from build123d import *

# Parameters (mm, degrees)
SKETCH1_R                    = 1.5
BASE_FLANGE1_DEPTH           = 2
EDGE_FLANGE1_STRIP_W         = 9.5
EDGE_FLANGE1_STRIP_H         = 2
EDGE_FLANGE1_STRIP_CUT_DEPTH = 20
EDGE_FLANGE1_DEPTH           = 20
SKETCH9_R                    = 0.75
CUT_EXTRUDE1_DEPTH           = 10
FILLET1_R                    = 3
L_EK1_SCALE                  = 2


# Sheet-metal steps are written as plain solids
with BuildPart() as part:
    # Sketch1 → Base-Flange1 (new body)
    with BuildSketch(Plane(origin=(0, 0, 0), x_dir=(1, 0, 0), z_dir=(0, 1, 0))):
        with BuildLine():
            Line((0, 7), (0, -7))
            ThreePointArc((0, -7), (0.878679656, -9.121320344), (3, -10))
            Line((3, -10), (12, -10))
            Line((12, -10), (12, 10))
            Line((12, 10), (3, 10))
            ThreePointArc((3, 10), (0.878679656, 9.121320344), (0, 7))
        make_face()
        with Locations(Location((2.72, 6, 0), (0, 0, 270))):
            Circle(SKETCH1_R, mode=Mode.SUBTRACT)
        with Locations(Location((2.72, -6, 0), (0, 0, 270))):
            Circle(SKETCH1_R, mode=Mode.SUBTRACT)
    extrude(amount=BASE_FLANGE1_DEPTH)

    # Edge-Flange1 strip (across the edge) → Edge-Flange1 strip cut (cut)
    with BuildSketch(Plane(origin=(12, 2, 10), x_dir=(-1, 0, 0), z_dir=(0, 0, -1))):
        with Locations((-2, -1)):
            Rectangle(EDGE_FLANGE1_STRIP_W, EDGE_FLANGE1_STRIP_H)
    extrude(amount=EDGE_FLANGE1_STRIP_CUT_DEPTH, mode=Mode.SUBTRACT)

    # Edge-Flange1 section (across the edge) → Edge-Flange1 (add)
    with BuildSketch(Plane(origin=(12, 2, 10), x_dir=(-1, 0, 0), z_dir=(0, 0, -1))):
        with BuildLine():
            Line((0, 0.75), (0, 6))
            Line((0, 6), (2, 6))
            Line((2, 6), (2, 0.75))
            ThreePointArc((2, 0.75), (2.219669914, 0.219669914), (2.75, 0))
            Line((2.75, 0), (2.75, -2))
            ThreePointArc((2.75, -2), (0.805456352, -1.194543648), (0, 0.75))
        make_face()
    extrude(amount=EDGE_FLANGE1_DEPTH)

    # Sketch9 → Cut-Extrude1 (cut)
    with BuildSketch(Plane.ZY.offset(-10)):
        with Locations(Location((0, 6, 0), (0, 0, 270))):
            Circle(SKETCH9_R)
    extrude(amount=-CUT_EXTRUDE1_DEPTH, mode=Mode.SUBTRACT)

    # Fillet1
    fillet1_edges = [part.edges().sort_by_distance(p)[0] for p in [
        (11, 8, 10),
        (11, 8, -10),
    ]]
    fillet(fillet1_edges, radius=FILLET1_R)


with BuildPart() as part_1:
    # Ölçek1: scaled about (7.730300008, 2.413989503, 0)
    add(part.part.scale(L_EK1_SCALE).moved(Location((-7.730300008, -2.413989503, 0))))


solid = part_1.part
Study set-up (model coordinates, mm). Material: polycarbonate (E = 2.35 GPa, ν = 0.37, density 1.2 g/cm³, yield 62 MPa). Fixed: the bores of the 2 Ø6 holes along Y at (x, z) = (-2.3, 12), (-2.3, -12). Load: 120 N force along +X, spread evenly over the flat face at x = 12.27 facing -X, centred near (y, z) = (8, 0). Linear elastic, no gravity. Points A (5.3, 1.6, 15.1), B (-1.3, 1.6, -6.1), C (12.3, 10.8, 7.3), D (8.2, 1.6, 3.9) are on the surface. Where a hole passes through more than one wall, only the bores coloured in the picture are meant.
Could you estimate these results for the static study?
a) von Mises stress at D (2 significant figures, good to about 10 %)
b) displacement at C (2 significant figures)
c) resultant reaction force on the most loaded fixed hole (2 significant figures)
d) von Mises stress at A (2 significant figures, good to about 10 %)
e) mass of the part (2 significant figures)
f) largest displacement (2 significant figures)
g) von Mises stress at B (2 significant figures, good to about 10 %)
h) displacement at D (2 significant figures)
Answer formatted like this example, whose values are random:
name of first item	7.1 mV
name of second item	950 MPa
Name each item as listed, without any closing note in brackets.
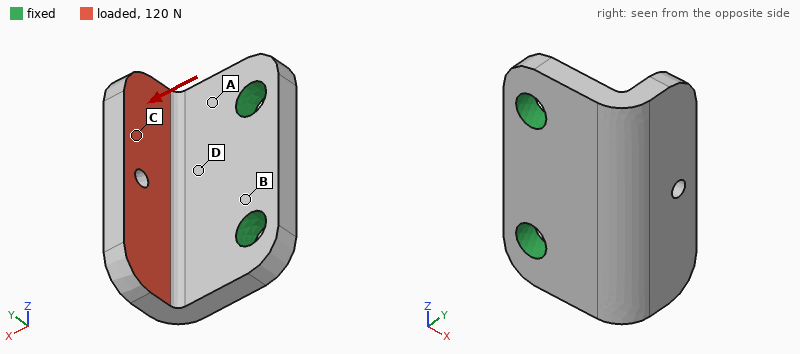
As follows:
von Mises stress at D	8.9 MPa
displacement at C	0.40 mm
resultant reaction force on the most loaded fixed hole	62 N
von Mises stress at A	10.0 MPa
mass of the part	6.2 g
largest displacement	0.55 mm
von Mises stress at B	4.6 MPa
displacement at D	0.096 mm
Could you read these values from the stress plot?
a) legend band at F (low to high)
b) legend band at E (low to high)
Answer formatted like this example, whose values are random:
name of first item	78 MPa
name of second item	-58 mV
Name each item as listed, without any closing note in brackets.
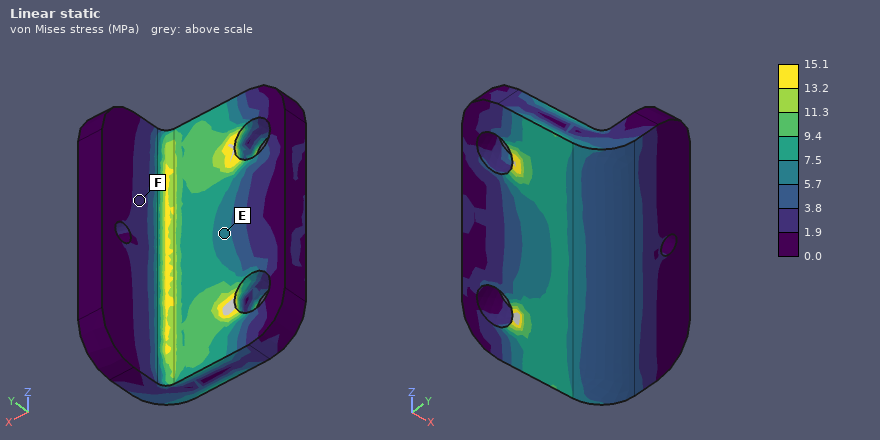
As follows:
legend band at F	1.9 to 3.8 MPa
legend band at E	5.7 to 7.5 MPa
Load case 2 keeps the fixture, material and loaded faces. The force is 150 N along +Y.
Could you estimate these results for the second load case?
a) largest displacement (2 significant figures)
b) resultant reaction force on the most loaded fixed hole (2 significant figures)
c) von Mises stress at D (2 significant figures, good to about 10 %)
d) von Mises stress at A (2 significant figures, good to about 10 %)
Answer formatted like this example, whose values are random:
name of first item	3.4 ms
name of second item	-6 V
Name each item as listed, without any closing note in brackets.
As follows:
largest displacement	0.46 mm
resultant reaction force on the most loaded fixed hole	75 N
von Mises stress at D	4.8 MPa
von Mises stress at A	9.8 MPa
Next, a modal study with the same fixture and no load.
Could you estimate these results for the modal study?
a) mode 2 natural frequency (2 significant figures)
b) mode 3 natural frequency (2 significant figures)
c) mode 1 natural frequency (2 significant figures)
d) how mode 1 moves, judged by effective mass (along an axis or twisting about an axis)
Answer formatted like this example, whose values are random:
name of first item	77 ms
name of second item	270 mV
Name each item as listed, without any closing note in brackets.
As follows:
mode 2 natural frequency	2400 Hz
mode 3 natural frequency	4300 Hz
mode 1 natural frequency	1500 Hz
how mode 1 moves, judged by effective mass	along Y
